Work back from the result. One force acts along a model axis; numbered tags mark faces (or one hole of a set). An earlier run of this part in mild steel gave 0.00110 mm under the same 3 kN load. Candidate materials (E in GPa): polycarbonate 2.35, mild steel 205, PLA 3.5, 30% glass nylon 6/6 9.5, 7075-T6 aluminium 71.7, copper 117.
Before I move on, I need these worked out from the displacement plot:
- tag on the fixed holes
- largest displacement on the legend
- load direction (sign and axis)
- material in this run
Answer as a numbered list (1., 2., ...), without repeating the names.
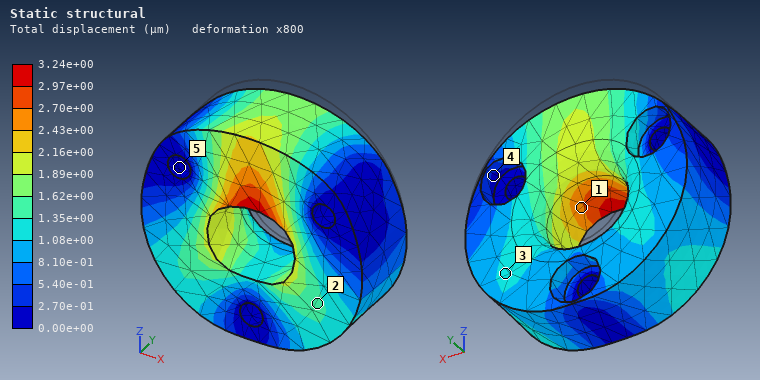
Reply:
1. 5
2. 3.24e+00 µm
3. -Z
4. 7075-T6 aluminium
